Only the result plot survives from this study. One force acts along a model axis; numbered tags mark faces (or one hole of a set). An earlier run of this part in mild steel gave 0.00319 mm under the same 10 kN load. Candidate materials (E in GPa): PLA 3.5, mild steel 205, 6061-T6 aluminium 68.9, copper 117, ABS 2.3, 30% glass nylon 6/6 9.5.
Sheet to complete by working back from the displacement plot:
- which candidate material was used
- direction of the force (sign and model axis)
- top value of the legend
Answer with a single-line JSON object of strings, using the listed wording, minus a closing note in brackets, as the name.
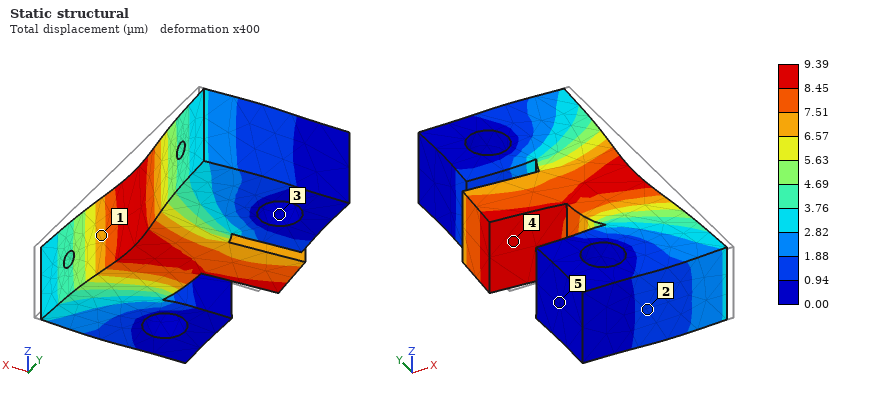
{"which candidate material was used": "6061-T6 aluminium", "direction of the force": "-X", "top value of the legend": "9.39 µm"}
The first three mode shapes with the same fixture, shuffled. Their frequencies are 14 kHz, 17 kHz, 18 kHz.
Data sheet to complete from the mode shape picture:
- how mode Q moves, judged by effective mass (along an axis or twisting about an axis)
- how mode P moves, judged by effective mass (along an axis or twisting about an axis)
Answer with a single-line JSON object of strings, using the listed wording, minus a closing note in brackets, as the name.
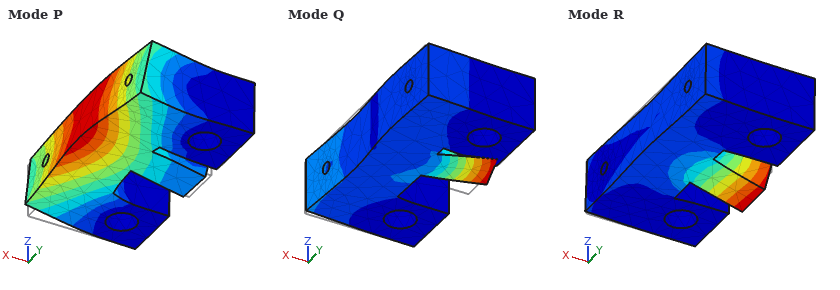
{"how mode Q moves, judged by effective mass": "along Y", "how mode P moves, judged by effective mass": "along Z"}
